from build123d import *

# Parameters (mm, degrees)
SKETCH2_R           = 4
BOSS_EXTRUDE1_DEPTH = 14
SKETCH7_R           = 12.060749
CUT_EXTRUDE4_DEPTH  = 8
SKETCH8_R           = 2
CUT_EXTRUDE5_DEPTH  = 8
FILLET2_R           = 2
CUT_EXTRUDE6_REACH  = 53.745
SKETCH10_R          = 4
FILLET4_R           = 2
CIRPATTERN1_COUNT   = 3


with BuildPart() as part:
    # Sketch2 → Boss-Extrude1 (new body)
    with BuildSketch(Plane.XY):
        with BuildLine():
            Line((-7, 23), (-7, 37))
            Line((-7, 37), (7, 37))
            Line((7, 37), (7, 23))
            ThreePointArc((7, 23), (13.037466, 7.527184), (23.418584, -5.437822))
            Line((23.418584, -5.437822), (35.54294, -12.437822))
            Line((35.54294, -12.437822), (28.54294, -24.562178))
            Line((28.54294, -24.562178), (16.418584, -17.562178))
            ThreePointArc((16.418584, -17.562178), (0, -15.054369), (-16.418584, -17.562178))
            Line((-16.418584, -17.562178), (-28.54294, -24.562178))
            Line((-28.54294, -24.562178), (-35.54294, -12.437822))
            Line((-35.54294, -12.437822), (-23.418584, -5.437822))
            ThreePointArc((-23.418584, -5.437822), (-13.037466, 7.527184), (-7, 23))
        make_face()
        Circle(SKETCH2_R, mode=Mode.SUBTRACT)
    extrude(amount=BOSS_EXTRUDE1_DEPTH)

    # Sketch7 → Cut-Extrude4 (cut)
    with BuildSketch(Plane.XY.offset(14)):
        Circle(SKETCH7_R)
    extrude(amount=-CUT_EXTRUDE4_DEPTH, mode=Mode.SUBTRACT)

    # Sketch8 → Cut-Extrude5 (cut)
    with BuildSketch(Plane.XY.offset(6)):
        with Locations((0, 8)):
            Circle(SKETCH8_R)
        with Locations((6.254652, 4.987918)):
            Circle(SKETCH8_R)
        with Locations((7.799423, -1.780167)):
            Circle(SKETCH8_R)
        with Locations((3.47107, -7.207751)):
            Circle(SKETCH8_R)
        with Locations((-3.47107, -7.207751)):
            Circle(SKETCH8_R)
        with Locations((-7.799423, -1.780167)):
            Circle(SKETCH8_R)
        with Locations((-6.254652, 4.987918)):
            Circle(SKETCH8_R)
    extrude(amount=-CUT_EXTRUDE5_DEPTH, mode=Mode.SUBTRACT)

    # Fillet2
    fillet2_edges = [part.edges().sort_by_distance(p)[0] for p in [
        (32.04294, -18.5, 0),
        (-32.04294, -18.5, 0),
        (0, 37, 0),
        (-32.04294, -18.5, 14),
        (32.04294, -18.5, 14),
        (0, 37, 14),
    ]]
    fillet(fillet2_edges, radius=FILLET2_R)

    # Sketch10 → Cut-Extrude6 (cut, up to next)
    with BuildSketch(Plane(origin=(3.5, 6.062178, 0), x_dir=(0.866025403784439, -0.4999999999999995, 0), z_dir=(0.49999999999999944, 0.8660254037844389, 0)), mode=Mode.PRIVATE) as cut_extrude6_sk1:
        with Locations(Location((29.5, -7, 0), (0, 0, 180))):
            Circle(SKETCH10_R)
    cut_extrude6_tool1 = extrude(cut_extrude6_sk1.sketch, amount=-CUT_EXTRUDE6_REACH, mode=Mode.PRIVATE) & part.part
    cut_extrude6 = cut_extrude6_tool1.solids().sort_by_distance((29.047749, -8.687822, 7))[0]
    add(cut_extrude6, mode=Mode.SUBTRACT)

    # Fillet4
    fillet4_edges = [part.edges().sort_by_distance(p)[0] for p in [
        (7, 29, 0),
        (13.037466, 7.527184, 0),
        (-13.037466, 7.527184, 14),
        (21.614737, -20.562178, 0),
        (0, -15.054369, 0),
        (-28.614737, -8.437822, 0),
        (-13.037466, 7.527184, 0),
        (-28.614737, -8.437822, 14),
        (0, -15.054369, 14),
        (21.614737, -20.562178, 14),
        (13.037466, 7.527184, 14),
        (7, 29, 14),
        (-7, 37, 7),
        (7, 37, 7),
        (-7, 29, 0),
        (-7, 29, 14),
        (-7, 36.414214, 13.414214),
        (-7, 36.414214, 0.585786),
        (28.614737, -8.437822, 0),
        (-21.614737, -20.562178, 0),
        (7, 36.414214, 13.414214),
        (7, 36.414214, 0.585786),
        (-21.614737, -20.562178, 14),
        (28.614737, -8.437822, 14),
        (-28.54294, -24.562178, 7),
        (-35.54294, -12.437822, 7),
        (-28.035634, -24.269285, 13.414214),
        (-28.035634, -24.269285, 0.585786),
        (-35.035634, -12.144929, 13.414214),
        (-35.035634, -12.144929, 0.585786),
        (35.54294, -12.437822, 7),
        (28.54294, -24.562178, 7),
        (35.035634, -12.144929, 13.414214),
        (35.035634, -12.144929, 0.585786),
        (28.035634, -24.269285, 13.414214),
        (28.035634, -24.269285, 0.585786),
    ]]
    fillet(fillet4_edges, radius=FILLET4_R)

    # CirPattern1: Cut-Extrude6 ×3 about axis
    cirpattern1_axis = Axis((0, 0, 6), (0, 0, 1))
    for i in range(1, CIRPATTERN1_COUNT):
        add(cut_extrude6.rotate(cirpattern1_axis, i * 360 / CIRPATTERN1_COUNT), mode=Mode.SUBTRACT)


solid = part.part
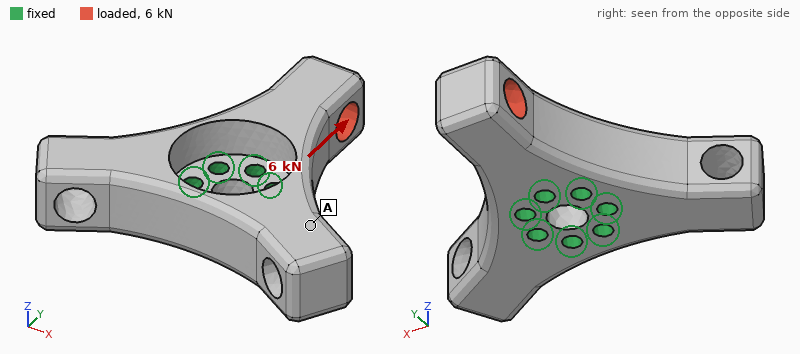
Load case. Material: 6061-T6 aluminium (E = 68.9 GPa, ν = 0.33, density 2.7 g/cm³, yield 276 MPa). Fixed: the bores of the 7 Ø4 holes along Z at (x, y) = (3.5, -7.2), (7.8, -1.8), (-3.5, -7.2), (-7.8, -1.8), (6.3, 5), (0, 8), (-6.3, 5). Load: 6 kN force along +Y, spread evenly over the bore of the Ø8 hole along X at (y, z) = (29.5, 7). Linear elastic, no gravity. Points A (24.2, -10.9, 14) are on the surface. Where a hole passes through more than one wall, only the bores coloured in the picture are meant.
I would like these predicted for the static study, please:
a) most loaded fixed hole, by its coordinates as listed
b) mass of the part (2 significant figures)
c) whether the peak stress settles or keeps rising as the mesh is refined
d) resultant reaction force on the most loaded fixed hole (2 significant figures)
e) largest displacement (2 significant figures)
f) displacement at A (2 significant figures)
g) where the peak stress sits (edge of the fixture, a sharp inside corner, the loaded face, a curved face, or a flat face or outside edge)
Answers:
(0, 8)
48 g
keeps rising
2.0 kN
58 µm
12 µm
edge of the fixture
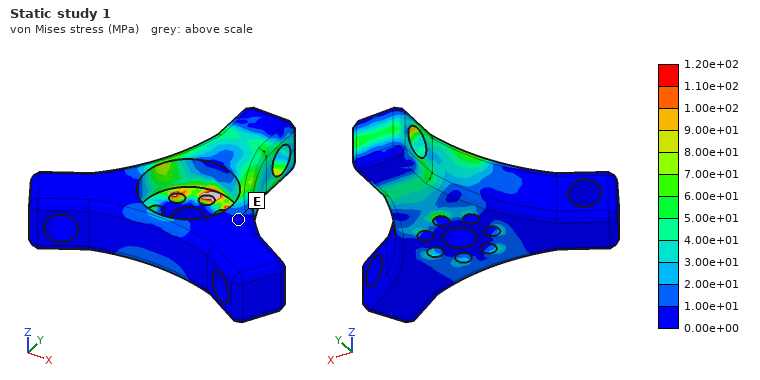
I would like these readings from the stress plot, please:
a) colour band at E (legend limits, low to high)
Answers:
0.00e+00 to 1.00e+01 MPa
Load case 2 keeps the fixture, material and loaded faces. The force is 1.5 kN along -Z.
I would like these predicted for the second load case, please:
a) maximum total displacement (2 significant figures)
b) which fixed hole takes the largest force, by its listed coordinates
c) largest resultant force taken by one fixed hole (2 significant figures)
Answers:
0.10 mm
(0, 8)
1.9 kN
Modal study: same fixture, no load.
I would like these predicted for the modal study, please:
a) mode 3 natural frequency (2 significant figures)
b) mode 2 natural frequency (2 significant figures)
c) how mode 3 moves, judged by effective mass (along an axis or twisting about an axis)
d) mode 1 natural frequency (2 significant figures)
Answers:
10 kHz
7700 Hz
along Z
7700 Hz
